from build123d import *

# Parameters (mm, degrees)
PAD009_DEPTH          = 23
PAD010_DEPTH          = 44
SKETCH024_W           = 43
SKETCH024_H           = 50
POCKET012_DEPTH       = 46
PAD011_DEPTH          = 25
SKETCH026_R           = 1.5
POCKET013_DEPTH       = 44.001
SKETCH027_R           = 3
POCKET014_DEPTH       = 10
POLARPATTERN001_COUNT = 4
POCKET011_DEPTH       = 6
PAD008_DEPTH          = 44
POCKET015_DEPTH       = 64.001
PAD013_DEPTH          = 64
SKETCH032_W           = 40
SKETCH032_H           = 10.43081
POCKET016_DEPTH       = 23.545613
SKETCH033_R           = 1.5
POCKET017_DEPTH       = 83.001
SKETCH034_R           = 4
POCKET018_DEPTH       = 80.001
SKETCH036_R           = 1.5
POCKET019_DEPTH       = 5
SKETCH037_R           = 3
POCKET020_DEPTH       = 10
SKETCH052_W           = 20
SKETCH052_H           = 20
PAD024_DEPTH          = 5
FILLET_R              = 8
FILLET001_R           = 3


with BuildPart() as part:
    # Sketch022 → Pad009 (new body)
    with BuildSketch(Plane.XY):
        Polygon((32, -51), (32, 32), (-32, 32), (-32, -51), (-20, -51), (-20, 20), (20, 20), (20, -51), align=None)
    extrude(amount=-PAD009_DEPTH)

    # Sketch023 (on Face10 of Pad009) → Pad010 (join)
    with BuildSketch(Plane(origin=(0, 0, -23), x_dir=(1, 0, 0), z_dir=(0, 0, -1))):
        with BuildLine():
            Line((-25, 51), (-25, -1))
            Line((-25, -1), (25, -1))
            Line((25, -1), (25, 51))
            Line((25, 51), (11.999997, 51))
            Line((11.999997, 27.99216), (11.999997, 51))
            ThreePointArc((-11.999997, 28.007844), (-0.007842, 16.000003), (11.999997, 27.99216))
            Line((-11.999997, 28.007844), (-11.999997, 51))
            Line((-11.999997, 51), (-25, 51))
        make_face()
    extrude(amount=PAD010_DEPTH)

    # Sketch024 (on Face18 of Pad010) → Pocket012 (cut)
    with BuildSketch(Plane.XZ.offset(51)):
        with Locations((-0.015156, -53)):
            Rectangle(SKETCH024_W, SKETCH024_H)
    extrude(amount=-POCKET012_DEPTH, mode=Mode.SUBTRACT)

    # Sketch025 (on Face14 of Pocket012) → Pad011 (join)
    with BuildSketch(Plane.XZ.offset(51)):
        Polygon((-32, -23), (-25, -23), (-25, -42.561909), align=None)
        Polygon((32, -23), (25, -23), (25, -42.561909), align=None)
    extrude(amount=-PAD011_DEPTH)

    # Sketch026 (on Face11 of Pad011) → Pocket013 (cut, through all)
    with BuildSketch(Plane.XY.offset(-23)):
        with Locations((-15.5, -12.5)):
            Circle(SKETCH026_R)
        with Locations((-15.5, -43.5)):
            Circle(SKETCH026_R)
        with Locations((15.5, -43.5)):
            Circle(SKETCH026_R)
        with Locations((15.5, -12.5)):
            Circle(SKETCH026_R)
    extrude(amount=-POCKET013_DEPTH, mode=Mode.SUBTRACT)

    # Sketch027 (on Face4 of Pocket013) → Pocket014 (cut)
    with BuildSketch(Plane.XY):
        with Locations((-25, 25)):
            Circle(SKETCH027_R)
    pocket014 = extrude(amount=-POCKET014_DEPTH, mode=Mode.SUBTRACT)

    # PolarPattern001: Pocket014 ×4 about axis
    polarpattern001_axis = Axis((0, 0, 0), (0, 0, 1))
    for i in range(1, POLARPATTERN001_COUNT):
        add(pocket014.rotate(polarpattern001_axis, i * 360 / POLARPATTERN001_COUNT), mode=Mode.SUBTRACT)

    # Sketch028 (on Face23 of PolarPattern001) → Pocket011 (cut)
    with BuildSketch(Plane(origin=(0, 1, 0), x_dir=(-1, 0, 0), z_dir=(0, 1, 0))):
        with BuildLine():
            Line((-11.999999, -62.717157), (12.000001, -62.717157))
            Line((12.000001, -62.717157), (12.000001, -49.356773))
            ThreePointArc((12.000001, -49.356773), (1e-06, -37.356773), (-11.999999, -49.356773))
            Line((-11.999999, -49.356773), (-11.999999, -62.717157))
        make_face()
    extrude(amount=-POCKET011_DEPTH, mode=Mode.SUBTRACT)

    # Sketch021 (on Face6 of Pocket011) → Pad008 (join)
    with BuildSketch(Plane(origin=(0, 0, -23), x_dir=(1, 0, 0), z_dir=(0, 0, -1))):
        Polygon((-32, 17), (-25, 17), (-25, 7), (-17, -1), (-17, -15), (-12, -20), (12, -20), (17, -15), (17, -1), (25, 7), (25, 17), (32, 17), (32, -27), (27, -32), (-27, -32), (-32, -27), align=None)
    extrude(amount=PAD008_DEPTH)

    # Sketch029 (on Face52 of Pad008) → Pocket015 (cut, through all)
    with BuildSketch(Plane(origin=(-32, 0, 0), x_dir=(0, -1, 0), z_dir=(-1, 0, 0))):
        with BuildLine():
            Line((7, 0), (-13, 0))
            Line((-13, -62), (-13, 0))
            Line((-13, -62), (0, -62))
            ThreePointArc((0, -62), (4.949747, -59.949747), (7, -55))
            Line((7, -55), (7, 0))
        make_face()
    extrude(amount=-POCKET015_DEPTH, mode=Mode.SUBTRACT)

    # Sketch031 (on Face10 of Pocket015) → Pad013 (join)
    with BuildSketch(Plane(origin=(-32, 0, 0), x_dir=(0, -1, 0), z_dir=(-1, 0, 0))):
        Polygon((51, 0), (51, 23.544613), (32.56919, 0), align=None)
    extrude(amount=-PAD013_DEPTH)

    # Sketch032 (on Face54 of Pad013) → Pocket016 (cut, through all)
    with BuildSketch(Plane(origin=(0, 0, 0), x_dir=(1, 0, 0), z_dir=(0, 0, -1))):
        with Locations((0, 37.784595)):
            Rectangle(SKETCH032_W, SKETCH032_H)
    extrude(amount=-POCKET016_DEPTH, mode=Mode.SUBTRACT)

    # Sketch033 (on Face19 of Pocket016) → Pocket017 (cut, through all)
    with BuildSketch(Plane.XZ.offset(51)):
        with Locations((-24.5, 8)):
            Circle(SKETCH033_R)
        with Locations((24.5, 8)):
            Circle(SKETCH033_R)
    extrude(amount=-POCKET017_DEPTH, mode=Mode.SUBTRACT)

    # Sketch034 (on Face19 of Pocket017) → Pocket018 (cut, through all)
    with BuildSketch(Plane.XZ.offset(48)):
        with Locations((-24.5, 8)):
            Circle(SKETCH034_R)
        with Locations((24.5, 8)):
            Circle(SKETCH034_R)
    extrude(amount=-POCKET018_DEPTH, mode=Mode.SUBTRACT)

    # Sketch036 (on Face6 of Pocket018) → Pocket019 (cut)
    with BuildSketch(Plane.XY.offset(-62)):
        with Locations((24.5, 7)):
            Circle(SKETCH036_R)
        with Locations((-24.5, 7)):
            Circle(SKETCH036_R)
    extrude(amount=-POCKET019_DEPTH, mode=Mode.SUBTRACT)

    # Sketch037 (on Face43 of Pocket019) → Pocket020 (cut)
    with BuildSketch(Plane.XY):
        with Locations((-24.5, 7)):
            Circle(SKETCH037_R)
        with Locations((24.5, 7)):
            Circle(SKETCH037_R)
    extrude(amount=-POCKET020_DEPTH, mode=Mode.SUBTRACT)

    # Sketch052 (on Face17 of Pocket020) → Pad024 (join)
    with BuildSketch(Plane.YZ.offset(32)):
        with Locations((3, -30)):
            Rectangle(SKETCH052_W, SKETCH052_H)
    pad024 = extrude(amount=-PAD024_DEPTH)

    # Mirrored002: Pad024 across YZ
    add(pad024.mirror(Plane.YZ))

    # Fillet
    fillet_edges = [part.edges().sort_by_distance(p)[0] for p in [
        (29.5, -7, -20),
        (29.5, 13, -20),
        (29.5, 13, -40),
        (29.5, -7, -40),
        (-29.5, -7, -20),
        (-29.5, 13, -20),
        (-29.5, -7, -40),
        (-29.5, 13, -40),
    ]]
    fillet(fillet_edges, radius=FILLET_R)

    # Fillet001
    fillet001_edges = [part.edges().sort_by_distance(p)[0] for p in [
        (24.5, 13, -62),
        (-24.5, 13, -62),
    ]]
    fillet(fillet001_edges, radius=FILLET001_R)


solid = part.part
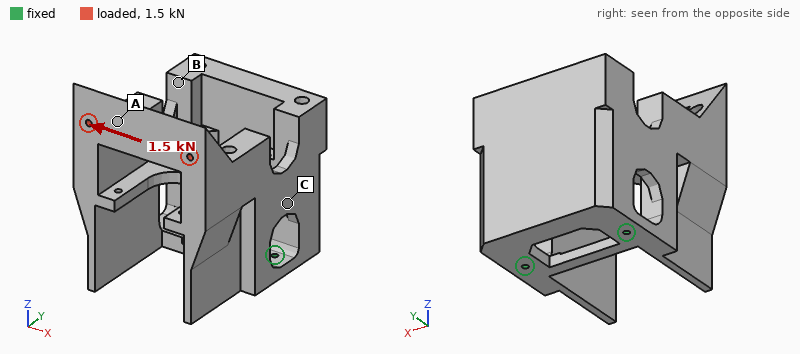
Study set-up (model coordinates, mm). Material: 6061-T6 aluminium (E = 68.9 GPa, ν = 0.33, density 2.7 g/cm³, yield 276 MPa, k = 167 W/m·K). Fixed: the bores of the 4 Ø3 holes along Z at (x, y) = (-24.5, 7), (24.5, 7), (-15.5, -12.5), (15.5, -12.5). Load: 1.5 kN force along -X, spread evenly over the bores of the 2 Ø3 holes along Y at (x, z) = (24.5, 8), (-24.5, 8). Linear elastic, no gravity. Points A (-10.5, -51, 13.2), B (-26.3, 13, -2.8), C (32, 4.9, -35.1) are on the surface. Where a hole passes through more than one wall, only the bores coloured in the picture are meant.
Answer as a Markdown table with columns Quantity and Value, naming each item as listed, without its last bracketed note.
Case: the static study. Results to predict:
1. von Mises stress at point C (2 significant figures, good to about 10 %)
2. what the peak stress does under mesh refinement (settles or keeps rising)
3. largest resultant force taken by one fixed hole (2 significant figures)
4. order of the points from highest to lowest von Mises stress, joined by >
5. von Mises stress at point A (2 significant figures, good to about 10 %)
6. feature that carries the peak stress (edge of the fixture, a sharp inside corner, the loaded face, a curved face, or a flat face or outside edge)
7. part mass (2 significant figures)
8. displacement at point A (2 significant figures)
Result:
| Quantity | Value |
|---|---|
| von Mises stress at point C | 11 MPa |
| what the peak stress does under mesh refinement | keeps rising |
| largest resultant force taken by one fixed hole | 1.2 kN |
| order of the points from highest to lowest von Mises stress, joined by > | A > C > B |
| von Mises stress at point A | 19 MPa |
| feature that carries the peak stress | edge of the fixture |
| part mass | 360 g |
| displacement at point A | 0.094 mm |
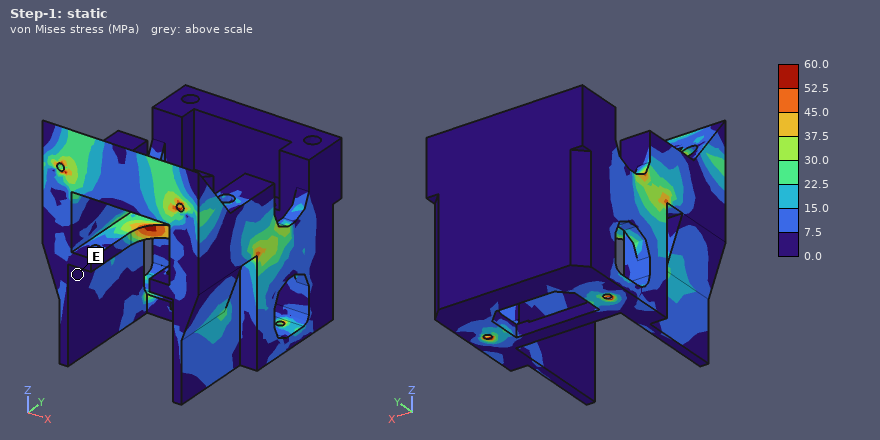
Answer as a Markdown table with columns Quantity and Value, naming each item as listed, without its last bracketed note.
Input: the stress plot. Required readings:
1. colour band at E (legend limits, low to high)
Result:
| Quantity | Value |
|---|---|
| colour band at E | 0.0 to 7.5 MPa |
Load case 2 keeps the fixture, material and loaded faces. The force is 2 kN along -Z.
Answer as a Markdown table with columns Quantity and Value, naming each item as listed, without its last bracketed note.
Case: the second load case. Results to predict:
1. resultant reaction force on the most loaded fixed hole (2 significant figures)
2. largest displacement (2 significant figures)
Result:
| Quantity | Value |
|---|---|
| resultant reaction force on the most loaded fixed hole | 1.2 kN |
| largest displacement | 80 µm |
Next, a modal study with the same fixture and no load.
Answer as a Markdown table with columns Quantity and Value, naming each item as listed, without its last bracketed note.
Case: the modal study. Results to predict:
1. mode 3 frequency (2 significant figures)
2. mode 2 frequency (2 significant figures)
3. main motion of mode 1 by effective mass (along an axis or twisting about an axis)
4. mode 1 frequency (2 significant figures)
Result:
| Quantity | Value |
|---|---|
| mode 3 frequency | 2900 Hz |
| mode 2 frequency | 2800 Hz |
| main motion of mode 1 by effective mass | along Y |
| mode 1 frequency | 2400 Hz |
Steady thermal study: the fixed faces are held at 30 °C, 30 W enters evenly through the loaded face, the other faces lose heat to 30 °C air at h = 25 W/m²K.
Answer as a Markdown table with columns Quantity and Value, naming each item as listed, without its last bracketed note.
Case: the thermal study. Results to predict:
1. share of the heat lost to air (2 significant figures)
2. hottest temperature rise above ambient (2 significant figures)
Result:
| Quantity | Value |
|---|---|
| share of the heat lost to air | 20 % |
| hottest temperature rise above ambient | 26 K |
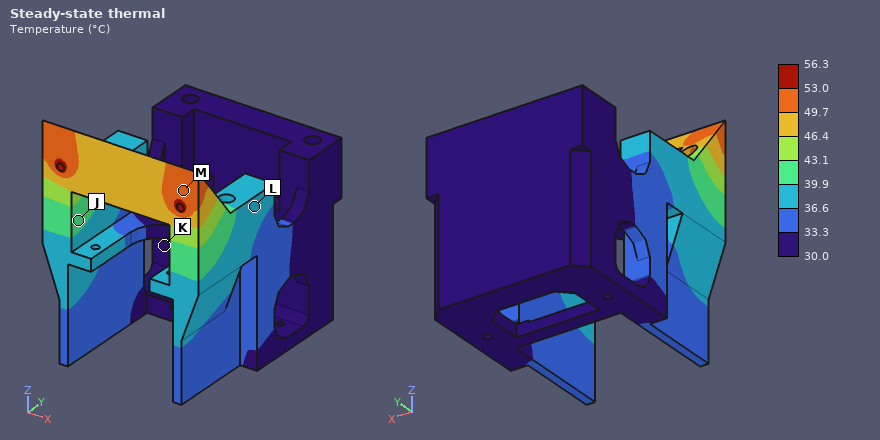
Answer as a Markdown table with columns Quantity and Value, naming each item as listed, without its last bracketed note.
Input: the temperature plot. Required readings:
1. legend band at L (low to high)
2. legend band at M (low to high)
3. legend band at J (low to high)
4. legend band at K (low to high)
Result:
| Quantity | Value |
|---|---|
| legend band at L | 36.6 to 39.9 °C |
| legend band at M | 49.7 to 53.0 °C |
| legend band at J | 39.9 to 43.1 °C |
| legend band at K | 30.0 to 33.3 °C |
